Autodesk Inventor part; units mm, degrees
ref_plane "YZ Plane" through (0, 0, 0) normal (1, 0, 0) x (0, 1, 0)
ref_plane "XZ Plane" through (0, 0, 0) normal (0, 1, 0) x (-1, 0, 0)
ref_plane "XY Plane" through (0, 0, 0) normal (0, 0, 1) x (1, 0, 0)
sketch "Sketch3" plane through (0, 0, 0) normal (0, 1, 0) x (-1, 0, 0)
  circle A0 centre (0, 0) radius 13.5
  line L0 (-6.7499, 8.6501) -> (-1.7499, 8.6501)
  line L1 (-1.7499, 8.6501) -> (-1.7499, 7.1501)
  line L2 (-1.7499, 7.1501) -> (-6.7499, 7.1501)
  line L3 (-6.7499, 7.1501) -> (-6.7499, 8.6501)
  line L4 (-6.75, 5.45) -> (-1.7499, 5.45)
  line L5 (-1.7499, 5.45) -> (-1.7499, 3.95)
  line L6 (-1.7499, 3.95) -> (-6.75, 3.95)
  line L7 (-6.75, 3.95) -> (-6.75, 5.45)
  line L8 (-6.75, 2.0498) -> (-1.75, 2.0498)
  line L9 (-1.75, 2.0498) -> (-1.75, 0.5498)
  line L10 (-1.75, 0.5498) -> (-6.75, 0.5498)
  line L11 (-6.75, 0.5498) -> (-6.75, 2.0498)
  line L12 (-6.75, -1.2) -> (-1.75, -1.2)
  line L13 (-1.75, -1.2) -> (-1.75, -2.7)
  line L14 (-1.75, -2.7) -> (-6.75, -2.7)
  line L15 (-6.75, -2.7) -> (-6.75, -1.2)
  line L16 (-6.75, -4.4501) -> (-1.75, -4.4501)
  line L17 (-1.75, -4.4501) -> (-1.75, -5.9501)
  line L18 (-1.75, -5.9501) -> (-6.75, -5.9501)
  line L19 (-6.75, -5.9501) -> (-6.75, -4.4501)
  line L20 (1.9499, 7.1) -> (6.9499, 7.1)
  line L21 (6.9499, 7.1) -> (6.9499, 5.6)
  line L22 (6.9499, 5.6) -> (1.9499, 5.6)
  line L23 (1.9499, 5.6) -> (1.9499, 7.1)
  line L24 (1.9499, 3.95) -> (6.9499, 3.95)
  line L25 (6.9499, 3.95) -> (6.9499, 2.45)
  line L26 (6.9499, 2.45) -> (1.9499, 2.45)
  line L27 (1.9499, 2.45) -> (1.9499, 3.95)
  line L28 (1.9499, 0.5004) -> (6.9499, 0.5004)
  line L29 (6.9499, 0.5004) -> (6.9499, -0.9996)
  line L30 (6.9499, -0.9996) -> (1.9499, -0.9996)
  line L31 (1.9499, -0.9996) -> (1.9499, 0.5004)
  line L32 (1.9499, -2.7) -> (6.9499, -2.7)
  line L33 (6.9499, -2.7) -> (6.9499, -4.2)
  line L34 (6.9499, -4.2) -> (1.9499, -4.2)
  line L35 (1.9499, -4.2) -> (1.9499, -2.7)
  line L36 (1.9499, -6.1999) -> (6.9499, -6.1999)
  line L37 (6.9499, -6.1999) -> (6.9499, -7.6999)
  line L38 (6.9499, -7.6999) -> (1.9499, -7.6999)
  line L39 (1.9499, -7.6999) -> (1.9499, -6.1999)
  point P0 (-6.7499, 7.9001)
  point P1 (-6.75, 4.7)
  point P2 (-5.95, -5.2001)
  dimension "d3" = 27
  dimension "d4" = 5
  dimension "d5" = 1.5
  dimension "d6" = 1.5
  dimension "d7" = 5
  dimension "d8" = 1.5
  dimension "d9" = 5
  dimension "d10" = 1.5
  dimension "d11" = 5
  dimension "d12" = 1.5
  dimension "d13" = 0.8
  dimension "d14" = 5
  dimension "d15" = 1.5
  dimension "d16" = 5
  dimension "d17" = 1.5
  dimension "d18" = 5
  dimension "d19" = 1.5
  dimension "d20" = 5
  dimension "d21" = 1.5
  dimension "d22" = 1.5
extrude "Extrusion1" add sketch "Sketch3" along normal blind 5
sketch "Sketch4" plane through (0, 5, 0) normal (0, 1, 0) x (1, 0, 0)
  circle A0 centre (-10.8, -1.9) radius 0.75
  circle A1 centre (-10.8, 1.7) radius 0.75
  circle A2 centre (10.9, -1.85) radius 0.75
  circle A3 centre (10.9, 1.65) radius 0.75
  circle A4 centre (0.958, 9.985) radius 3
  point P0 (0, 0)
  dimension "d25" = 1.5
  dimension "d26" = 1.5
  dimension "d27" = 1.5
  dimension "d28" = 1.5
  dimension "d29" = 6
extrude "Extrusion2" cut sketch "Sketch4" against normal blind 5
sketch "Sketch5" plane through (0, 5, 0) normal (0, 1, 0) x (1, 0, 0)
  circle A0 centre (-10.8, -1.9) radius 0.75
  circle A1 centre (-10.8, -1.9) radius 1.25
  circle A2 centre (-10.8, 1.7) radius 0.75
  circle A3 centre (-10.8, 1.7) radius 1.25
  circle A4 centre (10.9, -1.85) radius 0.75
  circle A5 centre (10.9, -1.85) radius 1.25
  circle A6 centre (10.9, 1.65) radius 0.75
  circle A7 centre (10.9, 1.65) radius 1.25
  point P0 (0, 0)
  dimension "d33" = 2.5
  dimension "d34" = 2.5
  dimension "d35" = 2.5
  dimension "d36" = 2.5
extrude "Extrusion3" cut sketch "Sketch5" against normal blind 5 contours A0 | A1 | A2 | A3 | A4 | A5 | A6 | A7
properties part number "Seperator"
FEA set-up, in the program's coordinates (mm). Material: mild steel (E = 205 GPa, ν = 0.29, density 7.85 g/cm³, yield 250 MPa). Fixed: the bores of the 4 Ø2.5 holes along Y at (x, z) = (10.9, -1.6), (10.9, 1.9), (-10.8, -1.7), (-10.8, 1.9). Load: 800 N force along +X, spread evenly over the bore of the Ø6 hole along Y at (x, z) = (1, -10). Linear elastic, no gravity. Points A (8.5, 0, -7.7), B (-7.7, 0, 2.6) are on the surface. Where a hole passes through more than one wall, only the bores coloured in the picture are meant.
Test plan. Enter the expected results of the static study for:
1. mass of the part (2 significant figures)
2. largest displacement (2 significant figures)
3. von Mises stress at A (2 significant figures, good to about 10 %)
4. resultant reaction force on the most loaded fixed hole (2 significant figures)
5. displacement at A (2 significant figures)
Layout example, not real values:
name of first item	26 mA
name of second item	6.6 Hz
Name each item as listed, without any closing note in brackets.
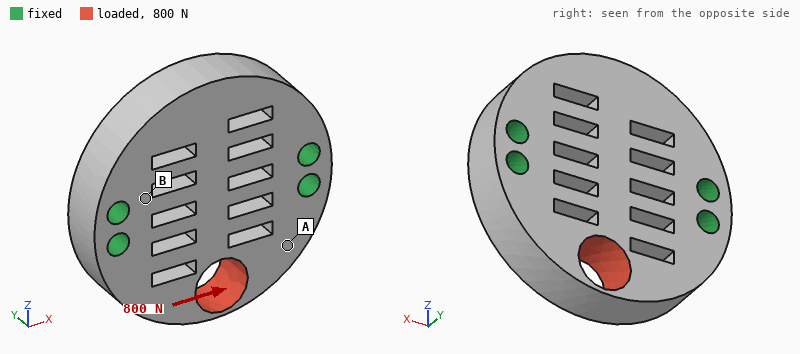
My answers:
mass of the part	18 g
largest displacement	3.3 µm
von Mises stress at A	11 MPa
resultant reaction force on the most loaded fixed hole	500 N
displacement at A	1.3 µm
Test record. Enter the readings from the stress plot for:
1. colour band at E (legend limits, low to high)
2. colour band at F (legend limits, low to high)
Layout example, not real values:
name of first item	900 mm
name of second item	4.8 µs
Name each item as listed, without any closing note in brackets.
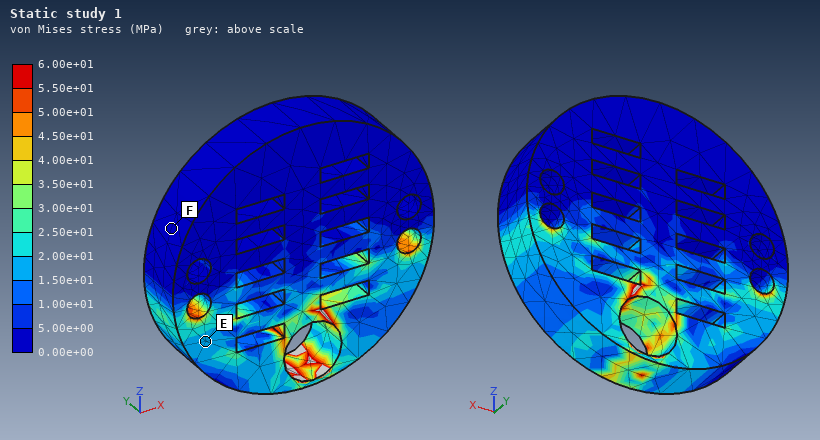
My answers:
colour band at E	1.50e+01 to 2.00e+01 MPa
colour band at F	0.00e+00 to 5.00e+00 MPa
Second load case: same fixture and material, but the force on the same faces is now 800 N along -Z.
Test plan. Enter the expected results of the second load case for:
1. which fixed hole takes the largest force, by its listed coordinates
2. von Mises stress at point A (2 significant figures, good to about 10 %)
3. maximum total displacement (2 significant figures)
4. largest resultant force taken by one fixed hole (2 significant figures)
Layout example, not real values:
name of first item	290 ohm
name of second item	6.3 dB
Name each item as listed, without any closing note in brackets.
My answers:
which fixed hole takes the largest force, by its listed coordinates	(10.9, -1.6)
von Mises stress at point A	10 MPa
maximum total displacement	3.2 µm
largest resultant force taken by one fixed hole	310 N
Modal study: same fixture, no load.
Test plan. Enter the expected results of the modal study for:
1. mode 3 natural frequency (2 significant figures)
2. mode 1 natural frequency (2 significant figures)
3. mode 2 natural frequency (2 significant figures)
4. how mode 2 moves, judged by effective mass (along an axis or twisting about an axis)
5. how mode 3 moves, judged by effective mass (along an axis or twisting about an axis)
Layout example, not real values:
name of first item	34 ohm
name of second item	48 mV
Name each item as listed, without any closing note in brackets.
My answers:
mode 3 natural frequency	42 kHz
mode 1 natural frequency	23 kHz
mode 2 natural frequency	26 kHz
how mode 2 moves, judged by effective mass	along Y
how mode 3 moves, judged by effective mass	along Z
